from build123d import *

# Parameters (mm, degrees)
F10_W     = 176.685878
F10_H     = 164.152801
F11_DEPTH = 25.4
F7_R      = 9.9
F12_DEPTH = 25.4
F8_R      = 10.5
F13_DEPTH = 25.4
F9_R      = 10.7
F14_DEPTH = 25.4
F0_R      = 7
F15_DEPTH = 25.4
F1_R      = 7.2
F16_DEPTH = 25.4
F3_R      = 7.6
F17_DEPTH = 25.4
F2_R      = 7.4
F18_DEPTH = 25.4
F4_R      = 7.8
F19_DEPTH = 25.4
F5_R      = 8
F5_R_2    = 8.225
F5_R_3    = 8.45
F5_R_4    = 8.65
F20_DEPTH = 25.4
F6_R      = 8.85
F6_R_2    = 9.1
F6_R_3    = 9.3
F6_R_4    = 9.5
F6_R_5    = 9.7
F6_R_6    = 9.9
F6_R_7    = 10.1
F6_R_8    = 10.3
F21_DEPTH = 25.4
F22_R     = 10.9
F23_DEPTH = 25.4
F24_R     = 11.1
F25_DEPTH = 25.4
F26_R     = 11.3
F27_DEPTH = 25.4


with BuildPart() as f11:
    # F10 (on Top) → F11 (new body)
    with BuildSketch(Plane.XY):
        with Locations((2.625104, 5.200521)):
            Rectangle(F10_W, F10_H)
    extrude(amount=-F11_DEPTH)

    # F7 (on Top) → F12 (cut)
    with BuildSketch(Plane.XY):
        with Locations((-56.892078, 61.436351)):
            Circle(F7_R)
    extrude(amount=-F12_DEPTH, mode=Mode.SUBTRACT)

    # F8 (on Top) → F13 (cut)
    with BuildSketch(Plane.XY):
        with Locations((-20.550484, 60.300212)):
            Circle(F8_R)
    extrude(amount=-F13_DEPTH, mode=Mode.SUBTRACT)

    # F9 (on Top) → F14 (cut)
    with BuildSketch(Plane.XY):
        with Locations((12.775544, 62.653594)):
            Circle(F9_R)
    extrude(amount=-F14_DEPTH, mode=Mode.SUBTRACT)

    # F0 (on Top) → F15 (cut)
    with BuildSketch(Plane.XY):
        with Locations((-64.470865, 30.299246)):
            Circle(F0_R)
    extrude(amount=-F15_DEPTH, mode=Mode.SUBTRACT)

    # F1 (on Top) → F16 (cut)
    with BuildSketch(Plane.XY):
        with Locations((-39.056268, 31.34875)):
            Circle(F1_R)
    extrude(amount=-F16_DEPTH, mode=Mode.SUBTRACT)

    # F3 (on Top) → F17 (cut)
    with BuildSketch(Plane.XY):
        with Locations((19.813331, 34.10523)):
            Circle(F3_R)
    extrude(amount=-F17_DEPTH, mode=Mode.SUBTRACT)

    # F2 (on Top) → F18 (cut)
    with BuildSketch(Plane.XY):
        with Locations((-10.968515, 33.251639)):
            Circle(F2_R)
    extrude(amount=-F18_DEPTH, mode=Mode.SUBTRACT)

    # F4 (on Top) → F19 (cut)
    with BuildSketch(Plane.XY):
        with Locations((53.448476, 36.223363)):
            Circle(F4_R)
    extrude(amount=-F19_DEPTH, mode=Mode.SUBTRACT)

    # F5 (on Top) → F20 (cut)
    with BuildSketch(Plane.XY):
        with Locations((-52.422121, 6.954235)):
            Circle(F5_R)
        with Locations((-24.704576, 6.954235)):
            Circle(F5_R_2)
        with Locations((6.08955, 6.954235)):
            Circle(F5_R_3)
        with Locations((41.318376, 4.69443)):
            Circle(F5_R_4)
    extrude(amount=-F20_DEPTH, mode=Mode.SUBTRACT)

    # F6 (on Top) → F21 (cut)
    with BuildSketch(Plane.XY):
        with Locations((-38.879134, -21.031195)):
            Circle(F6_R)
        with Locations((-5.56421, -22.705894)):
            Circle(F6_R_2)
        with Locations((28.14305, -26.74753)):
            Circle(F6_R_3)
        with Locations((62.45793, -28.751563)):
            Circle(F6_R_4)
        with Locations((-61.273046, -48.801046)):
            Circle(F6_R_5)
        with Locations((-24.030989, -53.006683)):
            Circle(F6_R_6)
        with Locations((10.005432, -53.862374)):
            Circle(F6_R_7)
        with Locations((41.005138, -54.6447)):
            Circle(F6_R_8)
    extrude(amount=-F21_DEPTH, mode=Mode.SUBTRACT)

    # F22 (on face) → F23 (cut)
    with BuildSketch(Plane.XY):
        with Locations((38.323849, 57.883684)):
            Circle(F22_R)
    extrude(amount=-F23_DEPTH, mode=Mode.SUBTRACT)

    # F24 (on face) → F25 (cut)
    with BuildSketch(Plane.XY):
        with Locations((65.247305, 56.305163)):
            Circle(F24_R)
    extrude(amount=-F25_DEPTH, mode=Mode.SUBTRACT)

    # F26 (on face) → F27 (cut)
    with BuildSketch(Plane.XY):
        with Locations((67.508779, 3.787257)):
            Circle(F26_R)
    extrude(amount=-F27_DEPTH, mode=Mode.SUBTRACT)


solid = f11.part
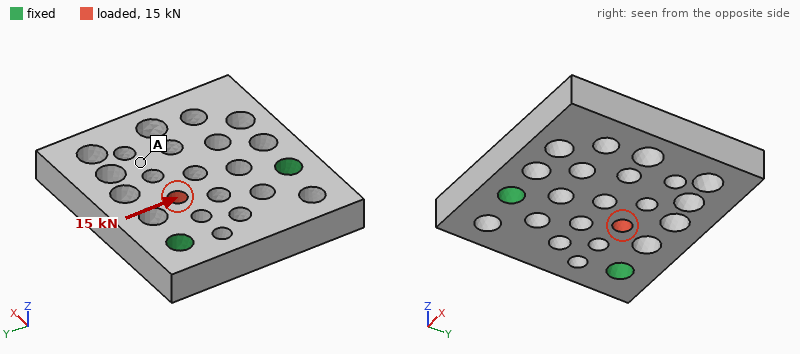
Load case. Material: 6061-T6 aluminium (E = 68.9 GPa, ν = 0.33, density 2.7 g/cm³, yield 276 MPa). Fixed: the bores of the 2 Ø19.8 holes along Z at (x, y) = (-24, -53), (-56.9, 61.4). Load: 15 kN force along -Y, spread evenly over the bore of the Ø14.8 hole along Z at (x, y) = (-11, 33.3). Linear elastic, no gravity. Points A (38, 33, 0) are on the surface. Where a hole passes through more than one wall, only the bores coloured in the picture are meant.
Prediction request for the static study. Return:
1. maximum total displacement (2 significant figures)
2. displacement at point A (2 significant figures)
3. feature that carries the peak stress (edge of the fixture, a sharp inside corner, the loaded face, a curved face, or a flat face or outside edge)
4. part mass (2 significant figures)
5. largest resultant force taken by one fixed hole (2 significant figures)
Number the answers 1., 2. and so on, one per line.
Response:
1. 16 µm
2. 9.8 µm
3. the loaded face
4. 1.6 kg
5. 8.2 kN
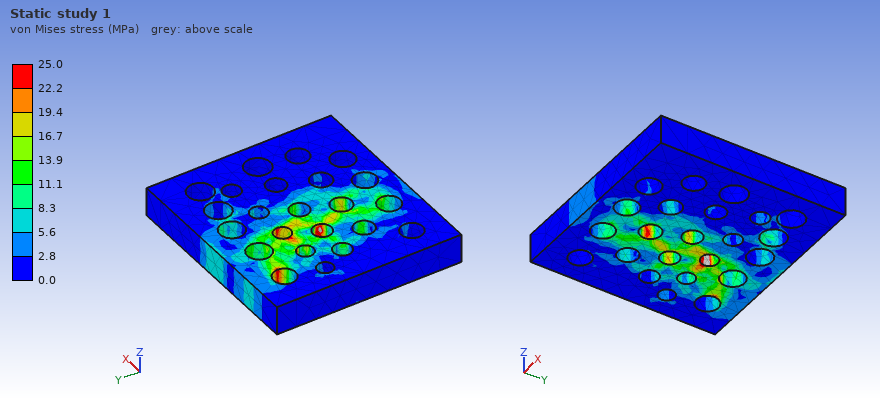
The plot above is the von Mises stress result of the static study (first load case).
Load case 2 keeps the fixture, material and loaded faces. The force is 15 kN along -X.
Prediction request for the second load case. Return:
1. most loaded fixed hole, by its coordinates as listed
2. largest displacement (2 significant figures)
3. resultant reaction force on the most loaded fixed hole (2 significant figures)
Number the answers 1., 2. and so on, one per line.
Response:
1. (-56.9, 61.4)
2. 14 µm
3. 12 kN
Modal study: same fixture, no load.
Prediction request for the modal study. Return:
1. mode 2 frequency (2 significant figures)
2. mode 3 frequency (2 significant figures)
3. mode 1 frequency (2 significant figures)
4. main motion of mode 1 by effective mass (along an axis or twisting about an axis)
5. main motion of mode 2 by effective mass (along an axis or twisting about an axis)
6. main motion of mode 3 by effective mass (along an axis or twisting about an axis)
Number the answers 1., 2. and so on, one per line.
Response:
1. 2000 Hz
2. 3700 Hz
3. 1000 Hz
4. along Z
5. twisting about X
6. along Y
